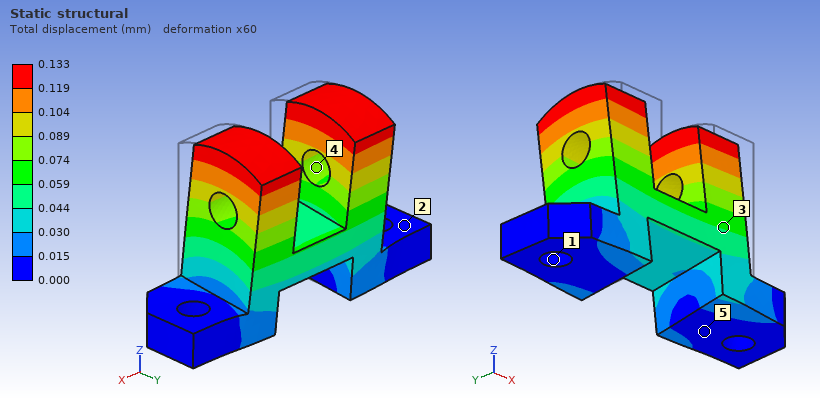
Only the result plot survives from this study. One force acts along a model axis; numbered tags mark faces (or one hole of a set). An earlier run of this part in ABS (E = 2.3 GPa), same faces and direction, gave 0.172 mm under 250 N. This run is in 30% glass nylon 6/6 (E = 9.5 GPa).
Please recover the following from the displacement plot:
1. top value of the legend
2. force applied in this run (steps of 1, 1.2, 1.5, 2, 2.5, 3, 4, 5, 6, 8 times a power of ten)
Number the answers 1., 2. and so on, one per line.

1. 0.133 mm
2. 800 N
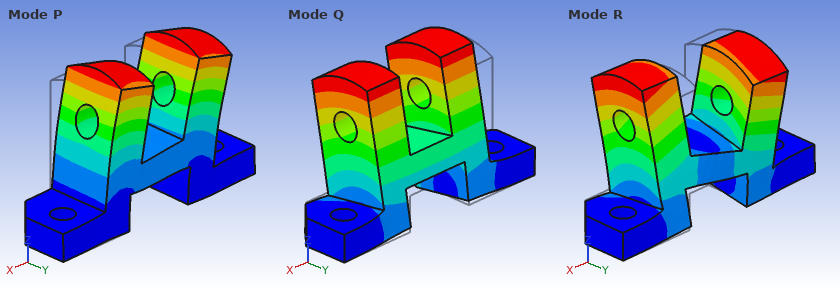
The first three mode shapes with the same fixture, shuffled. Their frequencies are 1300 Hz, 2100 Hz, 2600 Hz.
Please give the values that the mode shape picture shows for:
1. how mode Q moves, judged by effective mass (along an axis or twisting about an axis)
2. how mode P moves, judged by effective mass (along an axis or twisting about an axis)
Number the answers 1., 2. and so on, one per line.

1. along Y
2. along X
